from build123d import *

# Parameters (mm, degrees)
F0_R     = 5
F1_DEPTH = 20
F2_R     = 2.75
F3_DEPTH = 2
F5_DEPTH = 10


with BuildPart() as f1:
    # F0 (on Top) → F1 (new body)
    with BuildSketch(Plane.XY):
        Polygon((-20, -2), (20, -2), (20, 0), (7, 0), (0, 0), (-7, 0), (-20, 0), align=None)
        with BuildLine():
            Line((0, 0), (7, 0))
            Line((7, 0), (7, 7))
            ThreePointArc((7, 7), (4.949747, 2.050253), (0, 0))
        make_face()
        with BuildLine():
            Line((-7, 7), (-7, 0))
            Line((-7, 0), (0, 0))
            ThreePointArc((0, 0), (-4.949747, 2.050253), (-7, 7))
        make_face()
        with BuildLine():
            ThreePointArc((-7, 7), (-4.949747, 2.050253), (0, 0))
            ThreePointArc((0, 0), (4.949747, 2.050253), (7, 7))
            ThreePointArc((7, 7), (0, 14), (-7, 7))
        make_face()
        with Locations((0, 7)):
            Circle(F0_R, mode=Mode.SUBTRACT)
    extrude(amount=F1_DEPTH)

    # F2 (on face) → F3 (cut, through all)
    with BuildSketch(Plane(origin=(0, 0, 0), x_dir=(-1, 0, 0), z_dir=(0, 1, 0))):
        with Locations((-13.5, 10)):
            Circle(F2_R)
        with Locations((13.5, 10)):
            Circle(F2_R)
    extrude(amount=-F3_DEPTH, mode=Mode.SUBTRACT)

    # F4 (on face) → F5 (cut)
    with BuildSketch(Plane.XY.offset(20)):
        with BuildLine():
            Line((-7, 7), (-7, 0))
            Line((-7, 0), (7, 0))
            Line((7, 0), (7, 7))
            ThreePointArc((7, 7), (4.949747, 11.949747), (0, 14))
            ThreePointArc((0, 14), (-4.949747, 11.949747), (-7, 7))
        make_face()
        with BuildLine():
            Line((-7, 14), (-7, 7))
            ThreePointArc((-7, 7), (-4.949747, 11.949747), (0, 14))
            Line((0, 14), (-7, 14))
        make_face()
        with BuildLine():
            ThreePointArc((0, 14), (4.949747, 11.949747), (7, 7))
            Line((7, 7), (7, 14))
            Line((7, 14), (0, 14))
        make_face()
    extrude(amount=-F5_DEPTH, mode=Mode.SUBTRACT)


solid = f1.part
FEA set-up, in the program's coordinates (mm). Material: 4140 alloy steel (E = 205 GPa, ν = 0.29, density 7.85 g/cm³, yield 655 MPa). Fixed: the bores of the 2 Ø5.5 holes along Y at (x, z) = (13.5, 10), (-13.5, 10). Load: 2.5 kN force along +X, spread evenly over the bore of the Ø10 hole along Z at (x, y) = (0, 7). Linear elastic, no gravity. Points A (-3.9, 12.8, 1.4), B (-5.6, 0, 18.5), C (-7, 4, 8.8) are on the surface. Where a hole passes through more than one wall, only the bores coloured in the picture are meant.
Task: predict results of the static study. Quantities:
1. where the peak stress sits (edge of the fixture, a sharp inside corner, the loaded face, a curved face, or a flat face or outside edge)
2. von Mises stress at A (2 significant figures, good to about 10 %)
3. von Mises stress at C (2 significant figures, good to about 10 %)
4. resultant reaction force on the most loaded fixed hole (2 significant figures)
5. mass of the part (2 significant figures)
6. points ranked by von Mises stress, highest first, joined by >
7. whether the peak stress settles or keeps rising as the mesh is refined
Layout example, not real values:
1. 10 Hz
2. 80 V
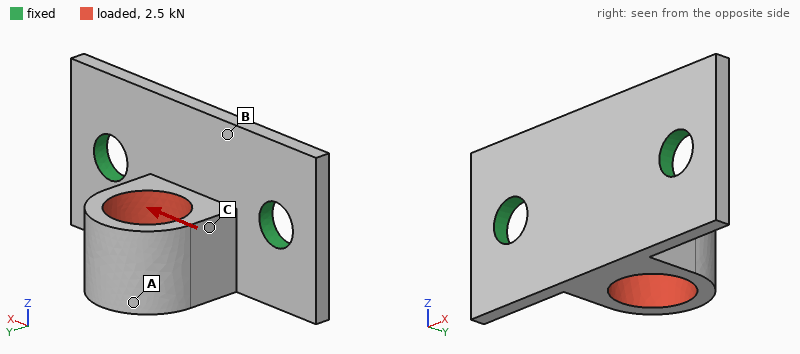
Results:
1. edge of the fixture
2. 110 MPa
3. 230 MPa
4. 1.7 kN
5. 19 g
6. C > A > B
7. keeps rising
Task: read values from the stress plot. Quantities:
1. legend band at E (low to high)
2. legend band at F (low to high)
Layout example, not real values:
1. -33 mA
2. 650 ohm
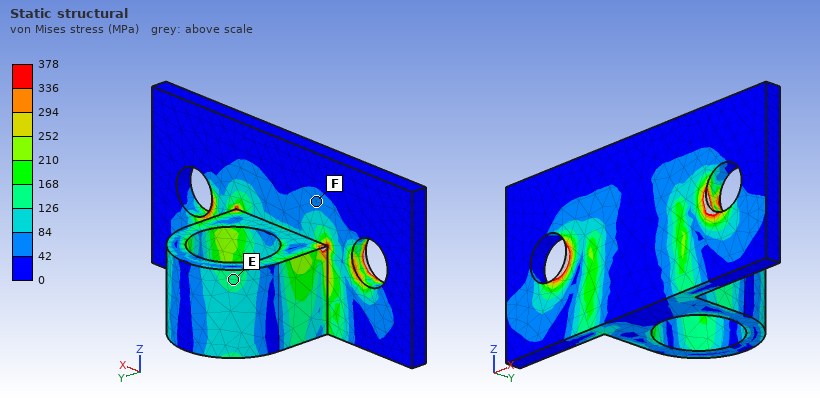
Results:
1. 126 to 168 MPa
2. 42 to 84 MPa
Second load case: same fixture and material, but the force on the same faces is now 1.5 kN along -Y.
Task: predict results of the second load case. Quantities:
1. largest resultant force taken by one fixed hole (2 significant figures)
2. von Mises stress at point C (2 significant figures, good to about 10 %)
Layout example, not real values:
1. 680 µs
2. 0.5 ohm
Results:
1. 830 N
2. 54 MPa
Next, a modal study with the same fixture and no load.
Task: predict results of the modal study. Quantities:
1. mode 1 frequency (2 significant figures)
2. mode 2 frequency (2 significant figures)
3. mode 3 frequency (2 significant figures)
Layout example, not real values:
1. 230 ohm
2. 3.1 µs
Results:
1. 6800 Hz
2. 15 kHz
3. 15 kHz
